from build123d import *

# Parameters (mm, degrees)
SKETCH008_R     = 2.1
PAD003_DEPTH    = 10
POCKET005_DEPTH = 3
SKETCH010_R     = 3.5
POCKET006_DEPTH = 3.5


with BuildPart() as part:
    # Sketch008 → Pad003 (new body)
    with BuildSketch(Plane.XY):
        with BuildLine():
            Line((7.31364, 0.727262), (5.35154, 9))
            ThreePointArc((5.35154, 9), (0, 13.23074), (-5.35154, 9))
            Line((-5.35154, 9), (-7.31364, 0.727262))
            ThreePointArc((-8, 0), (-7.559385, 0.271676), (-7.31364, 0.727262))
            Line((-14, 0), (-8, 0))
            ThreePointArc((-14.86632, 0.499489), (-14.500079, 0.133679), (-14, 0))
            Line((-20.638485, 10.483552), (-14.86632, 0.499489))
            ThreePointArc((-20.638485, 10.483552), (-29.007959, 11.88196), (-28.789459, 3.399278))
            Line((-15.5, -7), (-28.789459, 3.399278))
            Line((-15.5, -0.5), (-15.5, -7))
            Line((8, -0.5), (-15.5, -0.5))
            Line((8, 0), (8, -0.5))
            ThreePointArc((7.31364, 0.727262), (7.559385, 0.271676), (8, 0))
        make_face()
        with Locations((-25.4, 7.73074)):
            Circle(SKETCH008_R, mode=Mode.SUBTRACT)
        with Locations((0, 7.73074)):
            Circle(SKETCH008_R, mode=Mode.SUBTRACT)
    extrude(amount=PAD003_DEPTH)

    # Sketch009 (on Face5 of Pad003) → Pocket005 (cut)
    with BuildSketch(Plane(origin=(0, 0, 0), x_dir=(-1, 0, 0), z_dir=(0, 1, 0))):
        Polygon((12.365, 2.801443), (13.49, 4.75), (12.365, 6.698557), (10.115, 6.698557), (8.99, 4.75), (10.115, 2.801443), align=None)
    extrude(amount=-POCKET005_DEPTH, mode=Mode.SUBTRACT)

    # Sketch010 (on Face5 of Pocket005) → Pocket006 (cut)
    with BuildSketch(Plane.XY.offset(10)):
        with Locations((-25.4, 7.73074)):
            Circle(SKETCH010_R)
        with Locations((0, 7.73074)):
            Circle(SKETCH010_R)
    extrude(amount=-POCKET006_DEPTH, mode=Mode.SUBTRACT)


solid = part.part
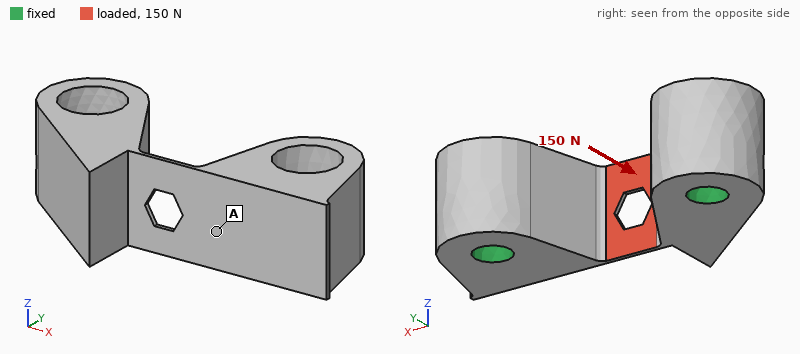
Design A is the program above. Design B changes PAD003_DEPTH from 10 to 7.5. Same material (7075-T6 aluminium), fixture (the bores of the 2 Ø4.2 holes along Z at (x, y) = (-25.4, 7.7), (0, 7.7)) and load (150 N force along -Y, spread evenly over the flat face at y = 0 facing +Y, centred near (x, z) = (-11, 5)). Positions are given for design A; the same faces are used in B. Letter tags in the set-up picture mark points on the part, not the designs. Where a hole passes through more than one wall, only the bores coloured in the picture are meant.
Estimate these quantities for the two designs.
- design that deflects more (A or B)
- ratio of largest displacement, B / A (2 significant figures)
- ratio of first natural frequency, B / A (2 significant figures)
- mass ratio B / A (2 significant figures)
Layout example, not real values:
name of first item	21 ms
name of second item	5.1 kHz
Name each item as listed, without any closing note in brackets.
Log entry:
design that deflects more	B
ratio of largest displacement, B / A	1.5
ratio of first natural frequency, B / A	1.1
mass ratio B / A	0.78
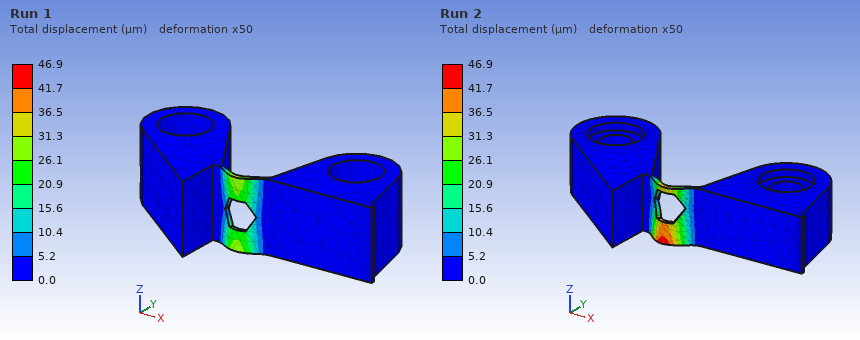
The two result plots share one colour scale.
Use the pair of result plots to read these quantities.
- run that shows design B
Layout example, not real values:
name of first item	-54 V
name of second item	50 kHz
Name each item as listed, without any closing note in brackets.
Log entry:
run that shows design B	Run 2
